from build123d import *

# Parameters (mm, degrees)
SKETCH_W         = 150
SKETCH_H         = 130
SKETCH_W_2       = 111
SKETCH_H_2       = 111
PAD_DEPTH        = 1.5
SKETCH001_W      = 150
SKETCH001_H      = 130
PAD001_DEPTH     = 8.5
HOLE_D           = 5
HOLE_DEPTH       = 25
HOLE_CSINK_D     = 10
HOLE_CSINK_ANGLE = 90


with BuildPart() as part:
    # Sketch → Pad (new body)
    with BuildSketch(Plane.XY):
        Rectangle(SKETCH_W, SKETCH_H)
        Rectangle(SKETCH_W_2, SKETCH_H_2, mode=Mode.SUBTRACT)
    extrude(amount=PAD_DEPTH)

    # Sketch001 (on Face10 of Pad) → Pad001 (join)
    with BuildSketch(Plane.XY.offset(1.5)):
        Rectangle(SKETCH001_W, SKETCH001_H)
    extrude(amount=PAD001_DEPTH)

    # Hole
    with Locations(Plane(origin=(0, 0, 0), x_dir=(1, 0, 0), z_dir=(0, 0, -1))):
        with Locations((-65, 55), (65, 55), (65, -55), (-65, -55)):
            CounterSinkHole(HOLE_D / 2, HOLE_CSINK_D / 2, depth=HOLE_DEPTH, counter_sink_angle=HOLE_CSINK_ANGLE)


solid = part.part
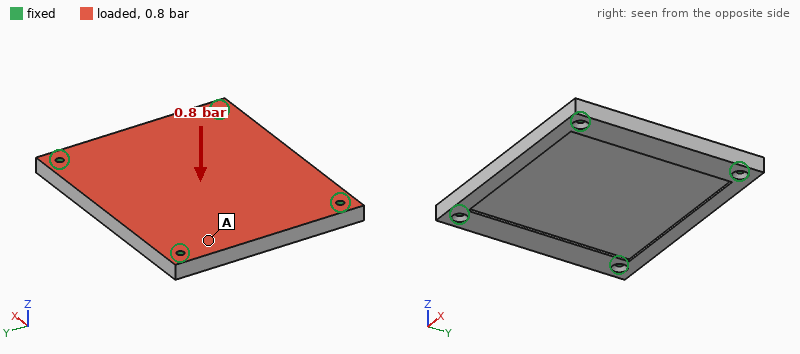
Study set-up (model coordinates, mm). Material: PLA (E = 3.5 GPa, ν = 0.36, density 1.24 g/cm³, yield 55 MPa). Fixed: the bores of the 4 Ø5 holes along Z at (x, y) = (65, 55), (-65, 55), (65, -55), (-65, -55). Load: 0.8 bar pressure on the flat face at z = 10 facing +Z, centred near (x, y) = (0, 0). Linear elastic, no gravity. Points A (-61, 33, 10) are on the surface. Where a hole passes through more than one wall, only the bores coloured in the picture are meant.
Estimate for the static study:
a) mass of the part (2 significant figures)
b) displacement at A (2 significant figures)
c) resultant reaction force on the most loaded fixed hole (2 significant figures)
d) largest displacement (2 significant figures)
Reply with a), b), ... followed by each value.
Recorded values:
a) 220 g
b) 0.18 mm
c) 390 N
d) 0.71 mm
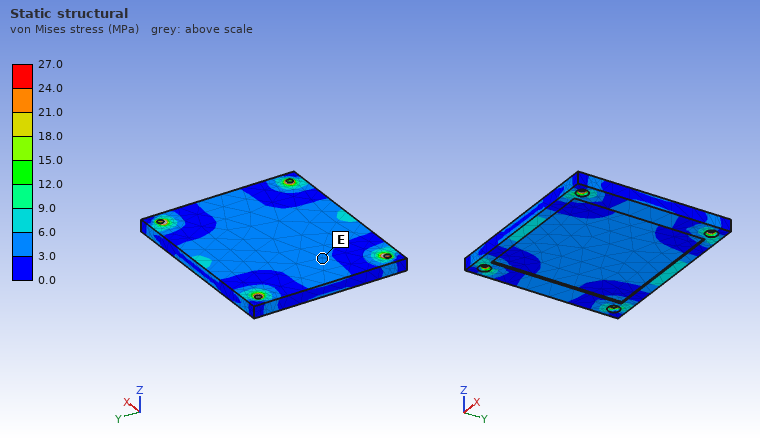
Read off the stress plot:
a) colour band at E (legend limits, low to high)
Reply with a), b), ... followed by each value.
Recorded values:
a) 3.0 to 6.0 MPa
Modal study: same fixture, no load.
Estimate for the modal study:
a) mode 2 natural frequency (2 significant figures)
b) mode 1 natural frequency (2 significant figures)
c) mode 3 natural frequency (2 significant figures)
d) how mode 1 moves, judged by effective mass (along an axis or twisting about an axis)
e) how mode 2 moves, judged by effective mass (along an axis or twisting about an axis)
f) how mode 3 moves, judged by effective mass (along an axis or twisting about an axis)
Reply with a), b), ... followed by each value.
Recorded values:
a) 980 Hz
b) 620 Hz
c) 1200 Hz
d) along Z
e) twisting about X
f) twisting about Y
